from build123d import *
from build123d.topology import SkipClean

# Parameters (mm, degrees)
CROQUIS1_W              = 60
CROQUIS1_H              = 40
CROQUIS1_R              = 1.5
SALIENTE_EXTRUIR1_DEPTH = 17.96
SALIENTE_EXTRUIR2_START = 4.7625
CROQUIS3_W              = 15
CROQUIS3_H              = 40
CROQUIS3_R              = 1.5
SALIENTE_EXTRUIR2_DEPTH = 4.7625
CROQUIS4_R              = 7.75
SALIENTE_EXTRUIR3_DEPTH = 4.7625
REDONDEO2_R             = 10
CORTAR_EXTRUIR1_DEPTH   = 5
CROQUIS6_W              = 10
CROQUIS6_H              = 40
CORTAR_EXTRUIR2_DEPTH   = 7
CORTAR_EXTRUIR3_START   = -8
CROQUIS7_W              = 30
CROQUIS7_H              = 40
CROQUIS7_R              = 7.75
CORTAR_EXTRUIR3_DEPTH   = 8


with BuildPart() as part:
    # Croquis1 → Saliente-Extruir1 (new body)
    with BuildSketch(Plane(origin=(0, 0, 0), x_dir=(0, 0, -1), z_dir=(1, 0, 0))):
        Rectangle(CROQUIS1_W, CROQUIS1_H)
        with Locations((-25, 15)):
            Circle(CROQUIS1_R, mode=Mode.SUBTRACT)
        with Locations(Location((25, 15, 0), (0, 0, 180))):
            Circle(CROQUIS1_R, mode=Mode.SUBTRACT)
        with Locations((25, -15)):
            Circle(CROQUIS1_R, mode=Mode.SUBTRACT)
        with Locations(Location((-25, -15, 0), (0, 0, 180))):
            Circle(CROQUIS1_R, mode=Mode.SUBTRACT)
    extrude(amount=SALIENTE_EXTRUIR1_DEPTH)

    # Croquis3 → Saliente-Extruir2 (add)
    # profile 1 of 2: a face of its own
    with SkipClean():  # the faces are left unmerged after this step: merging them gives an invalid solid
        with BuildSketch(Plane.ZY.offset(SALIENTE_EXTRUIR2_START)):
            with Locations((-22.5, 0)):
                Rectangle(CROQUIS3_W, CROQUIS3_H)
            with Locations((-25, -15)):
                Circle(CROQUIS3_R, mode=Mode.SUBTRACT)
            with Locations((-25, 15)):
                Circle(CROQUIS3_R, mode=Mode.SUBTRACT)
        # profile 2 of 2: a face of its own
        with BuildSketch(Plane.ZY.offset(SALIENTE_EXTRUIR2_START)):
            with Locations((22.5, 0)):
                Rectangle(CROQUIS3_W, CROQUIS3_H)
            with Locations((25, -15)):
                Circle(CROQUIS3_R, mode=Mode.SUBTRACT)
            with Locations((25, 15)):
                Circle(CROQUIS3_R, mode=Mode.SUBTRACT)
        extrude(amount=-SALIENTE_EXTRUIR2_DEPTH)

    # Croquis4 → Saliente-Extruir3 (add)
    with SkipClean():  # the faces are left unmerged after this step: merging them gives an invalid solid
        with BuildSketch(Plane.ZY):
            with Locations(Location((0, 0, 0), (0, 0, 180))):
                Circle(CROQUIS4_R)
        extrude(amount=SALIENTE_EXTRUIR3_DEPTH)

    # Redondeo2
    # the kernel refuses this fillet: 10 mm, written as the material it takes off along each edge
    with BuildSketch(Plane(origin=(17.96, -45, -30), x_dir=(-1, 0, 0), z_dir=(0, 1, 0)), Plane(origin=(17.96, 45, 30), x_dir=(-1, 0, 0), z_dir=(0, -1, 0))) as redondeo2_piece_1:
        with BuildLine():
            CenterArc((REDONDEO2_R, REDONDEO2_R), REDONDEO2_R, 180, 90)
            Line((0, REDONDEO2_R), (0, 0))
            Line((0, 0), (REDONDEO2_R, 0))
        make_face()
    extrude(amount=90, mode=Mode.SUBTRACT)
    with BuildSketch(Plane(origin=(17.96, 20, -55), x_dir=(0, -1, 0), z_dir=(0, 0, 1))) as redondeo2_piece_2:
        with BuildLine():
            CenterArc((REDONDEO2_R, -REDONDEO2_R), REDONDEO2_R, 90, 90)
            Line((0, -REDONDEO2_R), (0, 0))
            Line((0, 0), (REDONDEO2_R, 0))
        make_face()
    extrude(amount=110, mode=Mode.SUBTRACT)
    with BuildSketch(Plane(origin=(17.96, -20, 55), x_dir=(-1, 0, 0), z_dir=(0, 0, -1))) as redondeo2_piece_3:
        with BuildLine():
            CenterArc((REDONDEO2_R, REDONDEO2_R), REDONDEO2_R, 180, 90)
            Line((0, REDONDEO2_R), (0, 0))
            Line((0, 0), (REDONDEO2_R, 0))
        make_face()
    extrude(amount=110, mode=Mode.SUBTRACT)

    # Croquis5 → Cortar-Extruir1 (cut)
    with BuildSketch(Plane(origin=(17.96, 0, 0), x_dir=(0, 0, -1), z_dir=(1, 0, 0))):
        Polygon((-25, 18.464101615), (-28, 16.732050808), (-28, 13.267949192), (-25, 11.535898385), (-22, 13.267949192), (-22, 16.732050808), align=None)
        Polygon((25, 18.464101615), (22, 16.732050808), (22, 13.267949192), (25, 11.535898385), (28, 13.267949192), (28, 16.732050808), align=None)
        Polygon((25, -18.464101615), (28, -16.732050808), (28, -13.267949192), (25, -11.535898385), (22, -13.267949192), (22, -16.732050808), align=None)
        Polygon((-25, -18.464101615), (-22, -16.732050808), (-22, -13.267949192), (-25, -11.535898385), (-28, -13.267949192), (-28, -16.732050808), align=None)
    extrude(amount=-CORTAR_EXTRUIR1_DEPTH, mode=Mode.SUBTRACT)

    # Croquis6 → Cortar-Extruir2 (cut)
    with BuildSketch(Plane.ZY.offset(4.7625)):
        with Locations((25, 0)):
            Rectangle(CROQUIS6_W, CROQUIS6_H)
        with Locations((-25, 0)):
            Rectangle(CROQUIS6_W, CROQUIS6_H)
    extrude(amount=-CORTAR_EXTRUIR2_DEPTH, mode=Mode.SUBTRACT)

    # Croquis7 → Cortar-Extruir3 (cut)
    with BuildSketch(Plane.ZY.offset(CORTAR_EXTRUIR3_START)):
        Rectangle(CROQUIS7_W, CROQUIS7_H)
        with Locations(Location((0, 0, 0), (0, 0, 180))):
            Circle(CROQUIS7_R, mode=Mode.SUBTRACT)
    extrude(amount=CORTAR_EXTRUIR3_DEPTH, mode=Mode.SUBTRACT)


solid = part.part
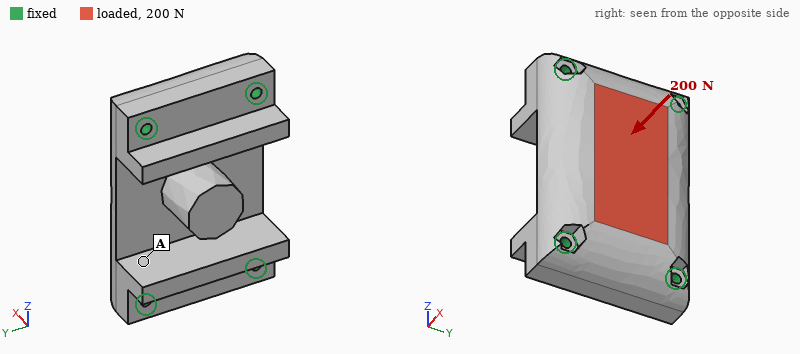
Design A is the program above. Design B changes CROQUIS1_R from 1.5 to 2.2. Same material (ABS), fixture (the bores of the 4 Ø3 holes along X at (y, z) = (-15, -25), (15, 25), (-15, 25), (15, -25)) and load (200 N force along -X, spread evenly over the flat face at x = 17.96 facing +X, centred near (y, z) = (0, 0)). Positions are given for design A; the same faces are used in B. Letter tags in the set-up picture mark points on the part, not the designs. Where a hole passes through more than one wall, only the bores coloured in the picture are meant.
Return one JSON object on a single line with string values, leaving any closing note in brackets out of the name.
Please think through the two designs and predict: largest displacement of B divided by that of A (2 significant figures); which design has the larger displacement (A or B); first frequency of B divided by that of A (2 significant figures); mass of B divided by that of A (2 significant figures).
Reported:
{"largest displacement of B divided by that of A": "0.90", "which design has the larger displacement": "A", "first frequency of B divided by that of A": "1.1", "mass of B divided by that of A": "0.99"}
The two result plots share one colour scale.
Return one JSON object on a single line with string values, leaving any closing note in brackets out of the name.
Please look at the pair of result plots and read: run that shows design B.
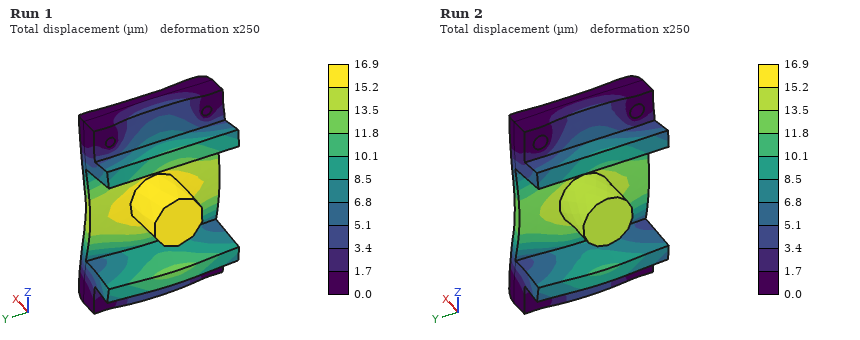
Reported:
{"run that shows design B": "Run 2"}
